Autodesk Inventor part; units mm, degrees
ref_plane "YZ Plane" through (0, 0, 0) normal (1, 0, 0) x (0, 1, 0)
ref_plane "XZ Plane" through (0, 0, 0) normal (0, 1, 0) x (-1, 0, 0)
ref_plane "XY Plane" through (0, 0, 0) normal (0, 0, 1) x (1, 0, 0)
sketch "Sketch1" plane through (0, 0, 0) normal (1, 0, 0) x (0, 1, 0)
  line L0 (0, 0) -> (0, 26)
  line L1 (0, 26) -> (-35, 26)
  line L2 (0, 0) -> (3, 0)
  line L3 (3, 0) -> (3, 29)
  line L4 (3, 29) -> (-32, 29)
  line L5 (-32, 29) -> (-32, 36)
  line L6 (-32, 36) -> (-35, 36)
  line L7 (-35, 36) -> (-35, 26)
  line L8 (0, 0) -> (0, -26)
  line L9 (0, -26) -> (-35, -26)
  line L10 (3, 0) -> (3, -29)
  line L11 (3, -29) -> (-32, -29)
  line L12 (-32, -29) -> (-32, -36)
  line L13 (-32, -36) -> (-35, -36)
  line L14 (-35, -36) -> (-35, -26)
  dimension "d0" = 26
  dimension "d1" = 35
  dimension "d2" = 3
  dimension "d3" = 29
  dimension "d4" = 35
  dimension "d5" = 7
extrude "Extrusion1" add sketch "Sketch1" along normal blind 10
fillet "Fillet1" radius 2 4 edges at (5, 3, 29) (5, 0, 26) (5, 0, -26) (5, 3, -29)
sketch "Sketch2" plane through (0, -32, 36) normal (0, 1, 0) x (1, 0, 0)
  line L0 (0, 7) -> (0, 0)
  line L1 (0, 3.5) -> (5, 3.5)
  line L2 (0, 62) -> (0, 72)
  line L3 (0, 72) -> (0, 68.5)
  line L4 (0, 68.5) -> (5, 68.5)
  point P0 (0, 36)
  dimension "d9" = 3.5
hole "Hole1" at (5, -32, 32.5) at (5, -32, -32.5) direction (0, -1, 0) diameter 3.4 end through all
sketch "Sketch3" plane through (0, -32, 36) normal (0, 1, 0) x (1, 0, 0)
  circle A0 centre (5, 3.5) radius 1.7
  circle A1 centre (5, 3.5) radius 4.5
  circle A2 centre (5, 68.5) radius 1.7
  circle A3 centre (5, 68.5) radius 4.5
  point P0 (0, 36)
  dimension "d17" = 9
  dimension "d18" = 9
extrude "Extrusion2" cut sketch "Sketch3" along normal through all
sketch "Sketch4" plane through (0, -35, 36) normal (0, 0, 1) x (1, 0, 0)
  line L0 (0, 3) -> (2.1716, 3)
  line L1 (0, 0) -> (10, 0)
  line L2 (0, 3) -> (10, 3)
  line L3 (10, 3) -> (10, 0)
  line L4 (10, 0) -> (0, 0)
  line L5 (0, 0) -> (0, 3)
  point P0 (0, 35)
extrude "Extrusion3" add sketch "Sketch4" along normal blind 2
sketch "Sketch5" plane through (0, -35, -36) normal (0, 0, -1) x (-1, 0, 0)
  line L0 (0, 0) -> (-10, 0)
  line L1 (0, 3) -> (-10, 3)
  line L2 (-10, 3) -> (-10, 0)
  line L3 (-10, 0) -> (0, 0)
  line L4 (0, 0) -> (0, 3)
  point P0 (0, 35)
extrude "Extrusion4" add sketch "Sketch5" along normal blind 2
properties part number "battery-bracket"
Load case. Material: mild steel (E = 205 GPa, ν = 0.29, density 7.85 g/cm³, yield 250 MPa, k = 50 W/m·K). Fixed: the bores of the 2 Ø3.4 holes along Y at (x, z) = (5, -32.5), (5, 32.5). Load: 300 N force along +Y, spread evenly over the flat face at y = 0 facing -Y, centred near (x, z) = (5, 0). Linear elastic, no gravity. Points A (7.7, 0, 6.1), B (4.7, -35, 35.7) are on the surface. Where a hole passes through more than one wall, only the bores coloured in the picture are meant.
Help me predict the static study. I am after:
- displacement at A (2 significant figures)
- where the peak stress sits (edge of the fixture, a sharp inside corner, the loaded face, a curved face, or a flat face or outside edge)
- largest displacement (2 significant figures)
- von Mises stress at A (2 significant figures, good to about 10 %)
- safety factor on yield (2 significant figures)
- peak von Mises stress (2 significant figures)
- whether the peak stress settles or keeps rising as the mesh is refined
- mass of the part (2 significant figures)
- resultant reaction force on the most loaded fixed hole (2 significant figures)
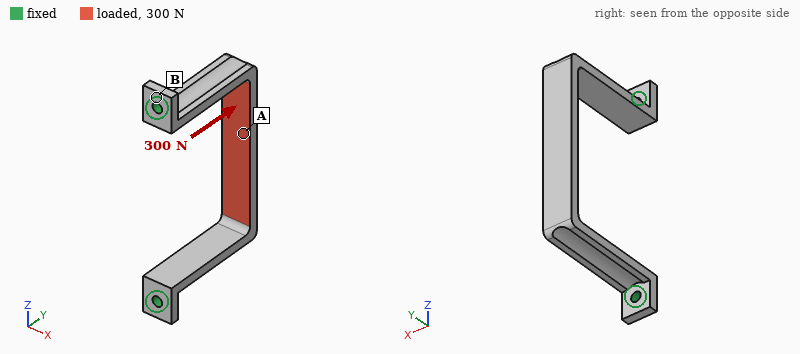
58 µm
a curved face
64 µm
66 MPa
2.5
100 MPa
settles
32 g
160 N
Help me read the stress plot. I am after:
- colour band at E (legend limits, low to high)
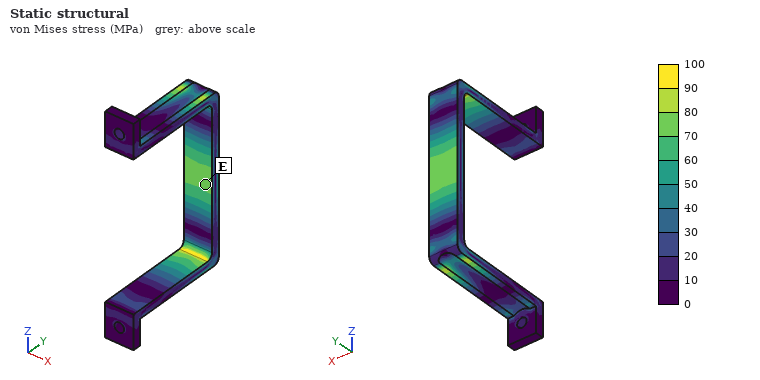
70 to 80 MPa
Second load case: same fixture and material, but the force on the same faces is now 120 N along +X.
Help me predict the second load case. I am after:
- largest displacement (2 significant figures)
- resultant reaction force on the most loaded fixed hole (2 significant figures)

58 µm
60 N
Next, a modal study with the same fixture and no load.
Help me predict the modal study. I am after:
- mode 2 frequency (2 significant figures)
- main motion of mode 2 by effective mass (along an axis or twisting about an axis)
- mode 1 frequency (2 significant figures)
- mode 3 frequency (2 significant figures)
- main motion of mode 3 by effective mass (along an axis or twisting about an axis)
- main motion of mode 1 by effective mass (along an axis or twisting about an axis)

1800 Hz
along X
1300 Hz
2800 Hz
twisting about Y
along Z
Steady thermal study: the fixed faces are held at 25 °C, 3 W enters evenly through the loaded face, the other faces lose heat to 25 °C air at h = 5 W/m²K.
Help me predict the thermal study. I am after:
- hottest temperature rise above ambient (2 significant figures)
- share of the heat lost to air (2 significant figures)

51 K
13 %
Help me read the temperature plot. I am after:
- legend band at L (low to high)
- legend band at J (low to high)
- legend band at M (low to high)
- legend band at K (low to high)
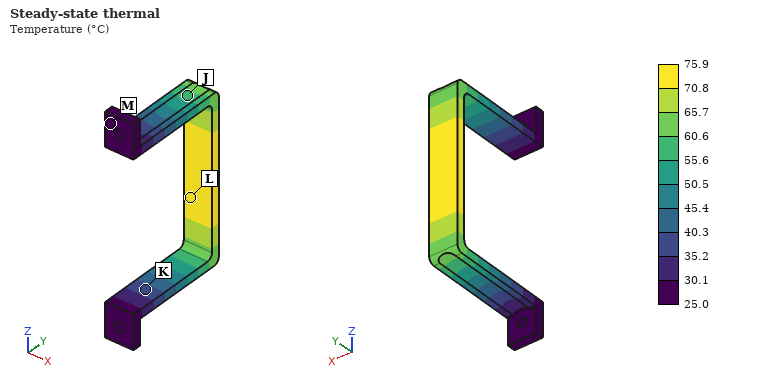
70.8 to 75.9 °C
55.6 to 60.6 °C
25.0 to 30.1 °C
35.2 to 40.3 °C
